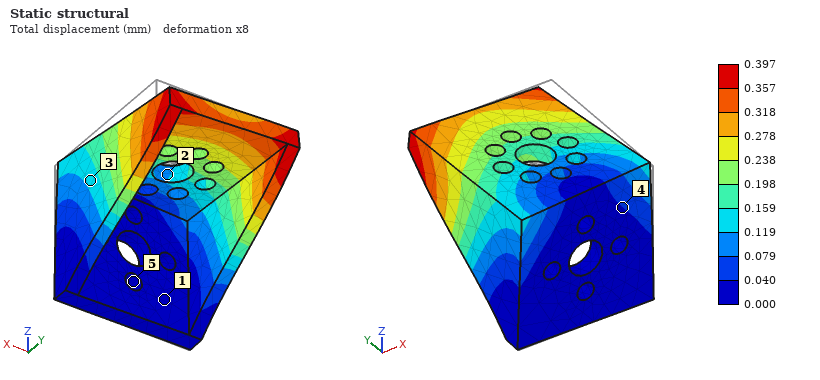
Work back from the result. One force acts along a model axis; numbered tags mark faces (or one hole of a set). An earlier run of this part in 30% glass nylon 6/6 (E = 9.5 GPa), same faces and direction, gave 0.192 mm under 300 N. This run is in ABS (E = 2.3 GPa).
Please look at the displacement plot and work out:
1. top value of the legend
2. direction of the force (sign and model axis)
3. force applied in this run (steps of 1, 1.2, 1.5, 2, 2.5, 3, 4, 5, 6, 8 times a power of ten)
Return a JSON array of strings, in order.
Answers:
["0.397 mm", "-X", "150 N"]
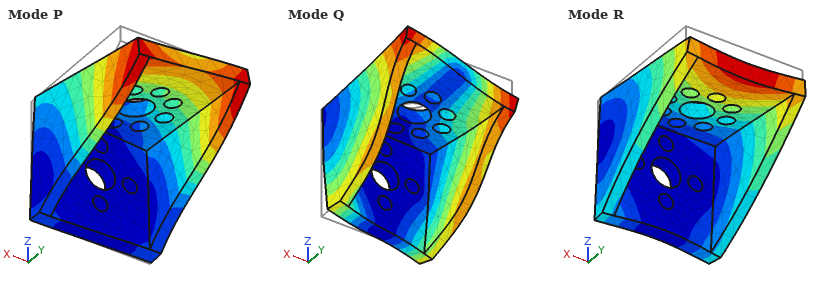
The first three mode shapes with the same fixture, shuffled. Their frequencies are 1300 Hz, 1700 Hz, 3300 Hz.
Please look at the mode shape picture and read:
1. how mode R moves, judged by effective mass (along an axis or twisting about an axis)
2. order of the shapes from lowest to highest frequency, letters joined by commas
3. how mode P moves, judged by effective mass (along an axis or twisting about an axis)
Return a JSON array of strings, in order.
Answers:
["along Z", "P, R, Q", "along X"]
